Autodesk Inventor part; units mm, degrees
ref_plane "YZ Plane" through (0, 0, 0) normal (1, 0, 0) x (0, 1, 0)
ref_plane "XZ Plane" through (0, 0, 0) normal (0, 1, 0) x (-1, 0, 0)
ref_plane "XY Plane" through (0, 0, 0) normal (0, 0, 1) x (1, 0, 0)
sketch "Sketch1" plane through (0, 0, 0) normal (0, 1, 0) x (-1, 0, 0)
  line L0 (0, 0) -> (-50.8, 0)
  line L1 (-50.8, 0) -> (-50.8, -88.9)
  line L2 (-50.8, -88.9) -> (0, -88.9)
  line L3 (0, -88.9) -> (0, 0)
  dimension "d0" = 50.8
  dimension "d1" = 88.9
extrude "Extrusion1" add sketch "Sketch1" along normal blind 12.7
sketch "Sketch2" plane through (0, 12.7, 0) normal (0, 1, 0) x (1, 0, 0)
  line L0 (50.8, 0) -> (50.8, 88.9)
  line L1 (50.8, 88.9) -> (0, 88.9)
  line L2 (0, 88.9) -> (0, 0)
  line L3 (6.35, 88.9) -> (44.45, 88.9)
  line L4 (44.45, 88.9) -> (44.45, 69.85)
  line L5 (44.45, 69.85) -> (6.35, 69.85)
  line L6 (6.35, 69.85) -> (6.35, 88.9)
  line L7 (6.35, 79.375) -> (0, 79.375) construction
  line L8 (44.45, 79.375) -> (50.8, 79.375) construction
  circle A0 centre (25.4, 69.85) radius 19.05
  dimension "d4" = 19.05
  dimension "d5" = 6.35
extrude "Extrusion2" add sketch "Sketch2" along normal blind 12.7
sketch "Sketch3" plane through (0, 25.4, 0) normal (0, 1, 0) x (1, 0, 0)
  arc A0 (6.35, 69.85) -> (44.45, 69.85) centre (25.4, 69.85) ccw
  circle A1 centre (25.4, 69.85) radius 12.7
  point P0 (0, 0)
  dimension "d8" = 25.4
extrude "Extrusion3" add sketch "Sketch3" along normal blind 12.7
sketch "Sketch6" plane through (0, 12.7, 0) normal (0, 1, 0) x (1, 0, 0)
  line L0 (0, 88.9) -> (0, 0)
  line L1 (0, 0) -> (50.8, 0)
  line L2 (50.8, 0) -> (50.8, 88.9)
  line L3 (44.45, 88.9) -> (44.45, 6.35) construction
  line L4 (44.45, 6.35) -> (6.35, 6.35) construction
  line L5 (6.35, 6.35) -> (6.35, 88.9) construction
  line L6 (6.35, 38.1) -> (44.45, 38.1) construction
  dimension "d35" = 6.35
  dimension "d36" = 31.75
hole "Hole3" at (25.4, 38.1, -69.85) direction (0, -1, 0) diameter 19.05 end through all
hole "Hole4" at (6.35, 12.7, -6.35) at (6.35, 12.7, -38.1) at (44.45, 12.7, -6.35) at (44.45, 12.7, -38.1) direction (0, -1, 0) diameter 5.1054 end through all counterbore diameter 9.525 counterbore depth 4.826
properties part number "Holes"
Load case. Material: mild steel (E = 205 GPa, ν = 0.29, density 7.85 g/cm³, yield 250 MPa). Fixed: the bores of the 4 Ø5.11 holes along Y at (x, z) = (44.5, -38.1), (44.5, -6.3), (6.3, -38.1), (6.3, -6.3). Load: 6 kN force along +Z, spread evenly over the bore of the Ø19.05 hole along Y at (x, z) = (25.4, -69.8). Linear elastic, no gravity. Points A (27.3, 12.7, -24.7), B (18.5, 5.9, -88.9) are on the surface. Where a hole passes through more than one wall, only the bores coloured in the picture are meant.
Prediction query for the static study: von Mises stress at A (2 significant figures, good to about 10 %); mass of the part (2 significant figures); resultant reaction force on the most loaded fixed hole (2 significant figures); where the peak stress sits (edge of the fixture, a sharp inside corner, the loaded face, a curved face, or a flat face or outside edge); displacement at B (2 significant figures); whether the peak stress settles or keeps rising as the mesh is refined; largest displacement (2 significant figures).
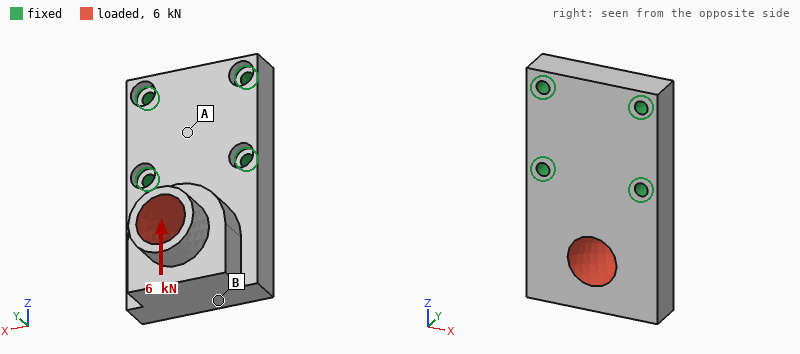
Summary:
24 MPa
530 g
1.8 kN
edge of the fixture
59 µm
keeps rising
71 µm
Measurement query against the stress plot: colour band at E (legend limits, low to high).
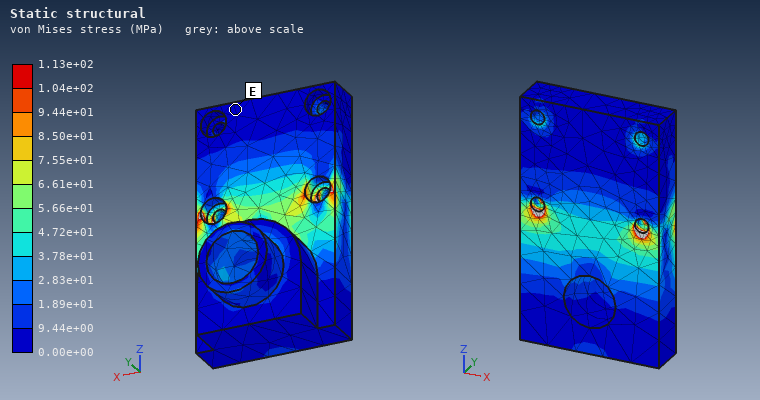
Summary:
0.00e+00 to 9.44e+00 MPa
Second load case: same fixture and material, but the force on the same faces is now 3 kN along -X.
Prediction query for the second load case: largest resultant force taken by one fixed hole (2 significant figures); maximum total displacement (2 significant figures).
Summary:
2.9 kN
12 µm
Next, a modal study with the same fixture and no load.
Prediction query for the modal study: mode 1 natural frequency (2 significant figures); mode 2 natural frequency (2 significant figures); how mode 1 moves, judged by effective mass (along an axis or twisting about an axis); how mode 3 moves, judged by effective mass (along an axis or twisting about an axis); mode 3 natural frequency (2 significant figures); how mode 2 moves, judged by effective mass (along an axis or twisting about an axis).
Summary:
2400 Hz
6500 Hz
along Y
along X
7400 Hz
along X
